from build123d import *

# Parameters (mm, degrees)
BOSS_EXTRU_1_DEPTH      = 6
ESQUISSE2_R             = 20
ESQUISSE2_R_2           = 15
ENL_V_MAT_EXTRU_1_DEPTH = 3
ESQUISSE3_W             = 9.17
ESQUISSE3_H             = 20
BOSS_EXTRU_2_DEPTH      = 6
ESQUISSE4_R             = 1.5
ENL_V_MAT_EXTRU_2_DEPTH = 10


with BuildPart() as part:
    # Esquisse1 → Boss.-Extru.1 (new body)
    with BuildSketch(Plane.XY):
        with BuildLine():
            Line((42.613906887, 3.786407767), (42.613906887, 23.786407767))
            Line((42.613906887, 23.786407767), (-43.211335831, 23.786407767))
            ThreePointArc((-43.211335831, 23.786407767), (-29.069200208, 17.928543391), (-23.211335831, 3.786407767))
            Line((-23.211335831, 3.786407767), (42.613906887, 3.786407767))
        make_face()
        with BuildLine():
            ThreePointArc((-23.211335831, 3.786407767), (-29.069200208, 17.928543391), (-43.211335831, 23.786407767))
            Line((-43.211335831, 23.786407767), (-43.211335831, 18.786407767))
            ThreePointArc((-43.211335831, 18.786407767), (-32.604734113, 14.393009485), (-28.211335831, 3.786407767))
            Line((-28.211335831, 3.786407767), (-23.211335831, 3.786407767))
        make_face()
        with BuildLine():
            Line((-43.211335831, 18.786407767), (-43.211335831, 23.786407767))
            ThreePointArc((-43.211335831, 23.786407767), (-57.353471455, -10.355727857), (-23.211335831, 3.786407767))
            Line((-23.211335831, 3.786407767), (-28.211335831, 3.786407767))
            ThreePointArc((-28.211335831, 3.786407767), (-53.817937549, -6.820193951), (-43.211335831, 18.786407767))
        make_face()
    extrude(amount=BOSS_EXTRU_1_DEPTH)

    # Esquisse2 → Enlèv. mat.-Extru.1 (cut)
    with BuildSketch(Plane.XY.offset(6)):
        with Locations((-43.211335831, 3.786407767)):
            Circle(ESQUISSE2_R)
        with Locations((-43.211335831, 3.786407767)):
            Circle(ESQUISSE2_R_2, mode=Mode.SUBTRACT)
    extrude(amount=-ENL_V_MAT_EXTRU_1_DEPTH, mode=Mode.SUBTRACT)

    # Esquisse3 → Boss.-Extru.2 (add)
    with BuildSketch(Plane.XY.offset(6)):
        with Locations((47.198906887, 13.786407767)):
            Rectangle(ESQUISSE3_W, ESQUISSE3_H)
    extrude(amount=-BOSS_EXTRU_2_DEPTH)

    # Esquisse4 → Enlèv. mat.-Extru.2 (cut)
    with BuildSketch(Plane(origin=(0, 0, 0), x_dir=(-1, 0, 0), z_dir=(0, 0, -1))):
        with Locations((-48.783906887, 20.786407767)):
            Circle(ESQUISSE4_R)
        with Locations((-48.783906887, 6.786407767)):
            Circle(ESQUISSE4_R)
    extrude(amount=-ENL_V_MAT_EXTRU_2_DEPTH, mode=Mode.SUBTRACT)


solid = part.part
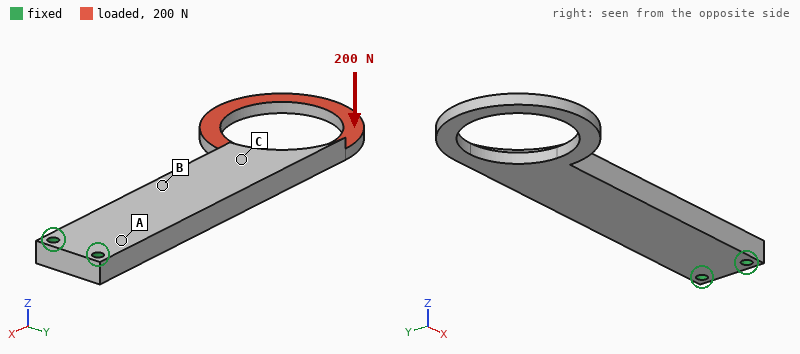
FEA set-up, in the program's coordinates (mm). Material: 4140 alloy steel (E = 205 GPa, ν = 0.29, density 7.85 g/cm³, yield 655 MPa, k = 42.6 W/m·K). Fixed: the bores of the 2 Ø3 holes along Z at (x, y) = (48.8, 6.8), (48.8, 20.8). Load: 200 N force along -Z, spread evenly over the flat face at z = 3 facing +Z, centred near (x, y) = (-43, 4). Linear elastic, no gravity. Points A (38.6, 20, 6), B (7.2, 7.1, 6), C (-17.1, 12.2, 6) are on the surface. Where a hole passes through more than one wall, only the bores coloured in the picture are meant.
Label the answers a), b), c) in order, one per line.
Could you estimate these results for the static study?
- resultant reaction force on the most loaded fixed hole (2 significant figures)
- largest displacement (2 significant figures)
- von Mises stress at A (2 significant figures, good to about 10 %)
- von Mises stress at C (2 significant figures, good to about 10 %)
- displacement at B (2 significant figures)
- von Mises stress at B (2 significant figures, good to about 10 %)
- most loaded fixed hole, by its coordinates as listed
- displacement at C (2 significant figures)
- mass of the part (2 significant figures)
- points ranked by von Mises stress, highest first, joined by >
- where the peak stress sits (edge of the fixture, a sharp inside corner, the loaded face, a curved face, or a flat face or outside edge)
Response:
a) 220 N
b) 1.3 mm
c) 140 MPa
d) 42 MPa
e) 0.19 mm
f) 87 MPa
g) (48.8, 6.8)
h) 0.42 mm
i) 87 g
j) A > B > C
k) a curved face
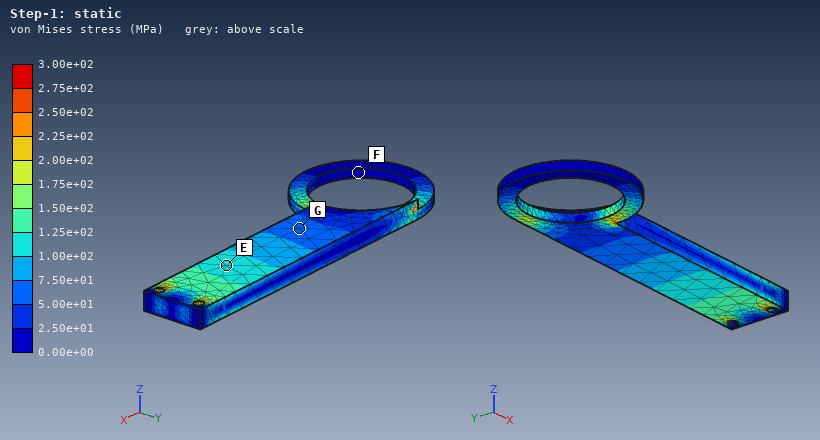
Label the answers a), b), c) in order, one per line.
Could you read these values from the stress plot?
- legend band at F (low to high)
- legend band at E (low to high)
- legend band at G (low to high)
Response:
a) 0.00e+00 to 2.50e+01 MPa
b) 1.00e+02 to 1.25e+02 MPa
c) 5.00e+01 to 7.50e+01 MPa
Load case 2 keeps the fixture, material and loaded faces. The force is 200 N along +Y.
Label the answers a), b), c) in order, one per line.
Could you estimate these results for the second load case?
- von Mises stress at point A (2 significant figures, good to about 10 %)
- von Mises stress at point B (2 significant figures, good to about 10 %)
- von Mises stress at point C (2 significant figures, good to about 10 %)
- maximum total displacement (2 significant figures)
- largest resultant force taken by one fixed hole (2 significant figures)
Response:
a) 26 MPa
b) 17 MPa
c) 8.3 MPa
d) 0.12 mm
e) 1.2 kN
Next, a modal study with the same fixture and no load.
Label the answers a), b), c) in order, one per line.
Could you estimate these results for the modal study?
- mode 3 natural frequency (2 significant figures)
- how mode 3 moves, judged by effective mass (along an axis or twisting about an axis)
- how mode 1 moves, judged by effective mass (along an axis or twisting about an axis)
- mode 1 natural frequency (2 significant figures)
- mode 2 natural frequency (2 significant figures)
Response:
a) 1700 Hz
b) along Y
c) along Z
d) 530 Hz
e) 1500 Hz
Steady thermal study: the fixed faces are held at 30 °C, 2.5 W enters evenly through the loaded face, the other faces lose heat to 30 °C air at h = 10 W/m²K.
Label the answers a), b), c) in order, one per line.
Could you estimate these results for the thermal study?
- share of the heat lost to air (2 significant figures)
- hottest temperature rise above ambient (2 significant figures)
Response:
a) 40 %
b) 55 K
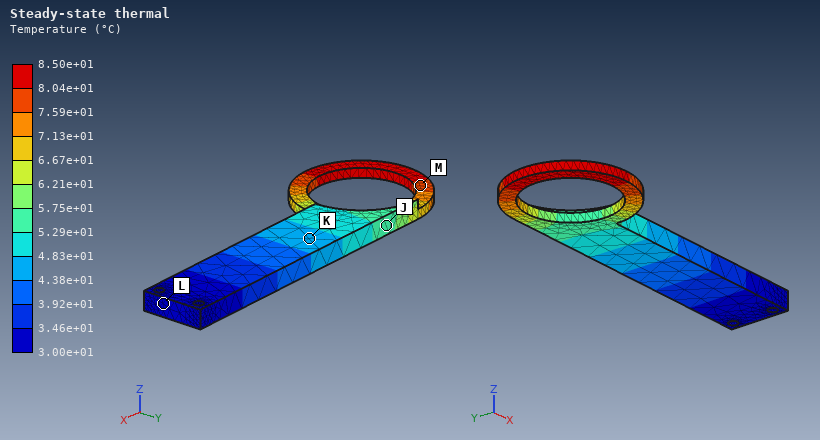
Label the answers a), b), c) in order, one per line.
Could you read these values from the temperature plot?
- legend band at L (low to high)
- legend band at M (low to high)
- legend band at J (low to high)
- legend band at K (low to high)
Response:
a) 3.00e+01 to 3.46e+01 °C
b) 7.59e+01 to 8.04e+01 °C
c) 5.29e+01 to 5.75e+01 °C
d) 4.38e+01 to 4.83e+01 °C
